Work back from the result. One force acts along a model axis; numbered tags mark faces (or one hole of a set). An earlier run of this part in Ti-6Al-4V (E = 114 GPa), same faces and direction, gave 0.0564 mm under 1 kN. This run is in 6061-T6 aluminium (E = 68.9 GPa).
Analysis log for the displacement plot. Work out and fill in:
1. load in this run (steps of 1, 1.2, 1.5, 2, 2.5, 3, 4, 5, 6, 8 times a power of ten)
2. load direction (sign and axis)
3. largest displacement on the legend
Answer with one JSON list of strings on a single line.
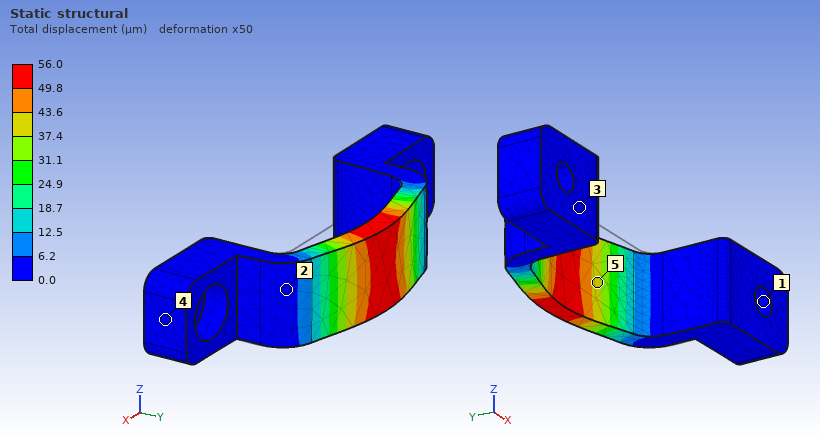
["600 N", "+Y", "56.0 µm"]
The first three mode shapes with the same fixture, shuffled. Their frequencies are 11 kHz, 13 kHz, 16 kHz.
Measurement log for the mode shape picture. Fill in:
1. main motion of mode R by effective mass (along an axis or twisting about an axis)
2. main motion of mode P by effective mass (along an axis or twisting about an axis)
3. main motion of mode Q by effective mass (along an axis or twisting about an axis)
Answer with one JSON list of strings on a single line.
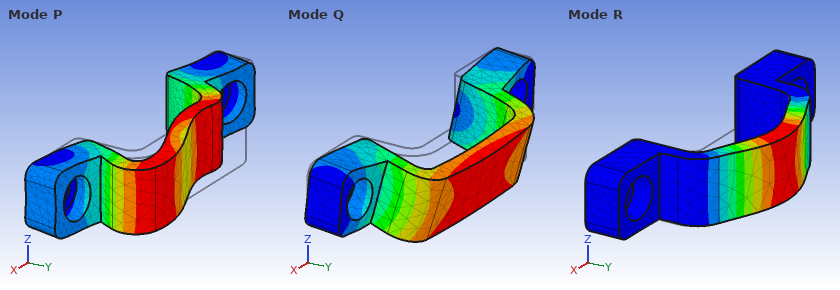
["along Y", "along X", "along Z"]
